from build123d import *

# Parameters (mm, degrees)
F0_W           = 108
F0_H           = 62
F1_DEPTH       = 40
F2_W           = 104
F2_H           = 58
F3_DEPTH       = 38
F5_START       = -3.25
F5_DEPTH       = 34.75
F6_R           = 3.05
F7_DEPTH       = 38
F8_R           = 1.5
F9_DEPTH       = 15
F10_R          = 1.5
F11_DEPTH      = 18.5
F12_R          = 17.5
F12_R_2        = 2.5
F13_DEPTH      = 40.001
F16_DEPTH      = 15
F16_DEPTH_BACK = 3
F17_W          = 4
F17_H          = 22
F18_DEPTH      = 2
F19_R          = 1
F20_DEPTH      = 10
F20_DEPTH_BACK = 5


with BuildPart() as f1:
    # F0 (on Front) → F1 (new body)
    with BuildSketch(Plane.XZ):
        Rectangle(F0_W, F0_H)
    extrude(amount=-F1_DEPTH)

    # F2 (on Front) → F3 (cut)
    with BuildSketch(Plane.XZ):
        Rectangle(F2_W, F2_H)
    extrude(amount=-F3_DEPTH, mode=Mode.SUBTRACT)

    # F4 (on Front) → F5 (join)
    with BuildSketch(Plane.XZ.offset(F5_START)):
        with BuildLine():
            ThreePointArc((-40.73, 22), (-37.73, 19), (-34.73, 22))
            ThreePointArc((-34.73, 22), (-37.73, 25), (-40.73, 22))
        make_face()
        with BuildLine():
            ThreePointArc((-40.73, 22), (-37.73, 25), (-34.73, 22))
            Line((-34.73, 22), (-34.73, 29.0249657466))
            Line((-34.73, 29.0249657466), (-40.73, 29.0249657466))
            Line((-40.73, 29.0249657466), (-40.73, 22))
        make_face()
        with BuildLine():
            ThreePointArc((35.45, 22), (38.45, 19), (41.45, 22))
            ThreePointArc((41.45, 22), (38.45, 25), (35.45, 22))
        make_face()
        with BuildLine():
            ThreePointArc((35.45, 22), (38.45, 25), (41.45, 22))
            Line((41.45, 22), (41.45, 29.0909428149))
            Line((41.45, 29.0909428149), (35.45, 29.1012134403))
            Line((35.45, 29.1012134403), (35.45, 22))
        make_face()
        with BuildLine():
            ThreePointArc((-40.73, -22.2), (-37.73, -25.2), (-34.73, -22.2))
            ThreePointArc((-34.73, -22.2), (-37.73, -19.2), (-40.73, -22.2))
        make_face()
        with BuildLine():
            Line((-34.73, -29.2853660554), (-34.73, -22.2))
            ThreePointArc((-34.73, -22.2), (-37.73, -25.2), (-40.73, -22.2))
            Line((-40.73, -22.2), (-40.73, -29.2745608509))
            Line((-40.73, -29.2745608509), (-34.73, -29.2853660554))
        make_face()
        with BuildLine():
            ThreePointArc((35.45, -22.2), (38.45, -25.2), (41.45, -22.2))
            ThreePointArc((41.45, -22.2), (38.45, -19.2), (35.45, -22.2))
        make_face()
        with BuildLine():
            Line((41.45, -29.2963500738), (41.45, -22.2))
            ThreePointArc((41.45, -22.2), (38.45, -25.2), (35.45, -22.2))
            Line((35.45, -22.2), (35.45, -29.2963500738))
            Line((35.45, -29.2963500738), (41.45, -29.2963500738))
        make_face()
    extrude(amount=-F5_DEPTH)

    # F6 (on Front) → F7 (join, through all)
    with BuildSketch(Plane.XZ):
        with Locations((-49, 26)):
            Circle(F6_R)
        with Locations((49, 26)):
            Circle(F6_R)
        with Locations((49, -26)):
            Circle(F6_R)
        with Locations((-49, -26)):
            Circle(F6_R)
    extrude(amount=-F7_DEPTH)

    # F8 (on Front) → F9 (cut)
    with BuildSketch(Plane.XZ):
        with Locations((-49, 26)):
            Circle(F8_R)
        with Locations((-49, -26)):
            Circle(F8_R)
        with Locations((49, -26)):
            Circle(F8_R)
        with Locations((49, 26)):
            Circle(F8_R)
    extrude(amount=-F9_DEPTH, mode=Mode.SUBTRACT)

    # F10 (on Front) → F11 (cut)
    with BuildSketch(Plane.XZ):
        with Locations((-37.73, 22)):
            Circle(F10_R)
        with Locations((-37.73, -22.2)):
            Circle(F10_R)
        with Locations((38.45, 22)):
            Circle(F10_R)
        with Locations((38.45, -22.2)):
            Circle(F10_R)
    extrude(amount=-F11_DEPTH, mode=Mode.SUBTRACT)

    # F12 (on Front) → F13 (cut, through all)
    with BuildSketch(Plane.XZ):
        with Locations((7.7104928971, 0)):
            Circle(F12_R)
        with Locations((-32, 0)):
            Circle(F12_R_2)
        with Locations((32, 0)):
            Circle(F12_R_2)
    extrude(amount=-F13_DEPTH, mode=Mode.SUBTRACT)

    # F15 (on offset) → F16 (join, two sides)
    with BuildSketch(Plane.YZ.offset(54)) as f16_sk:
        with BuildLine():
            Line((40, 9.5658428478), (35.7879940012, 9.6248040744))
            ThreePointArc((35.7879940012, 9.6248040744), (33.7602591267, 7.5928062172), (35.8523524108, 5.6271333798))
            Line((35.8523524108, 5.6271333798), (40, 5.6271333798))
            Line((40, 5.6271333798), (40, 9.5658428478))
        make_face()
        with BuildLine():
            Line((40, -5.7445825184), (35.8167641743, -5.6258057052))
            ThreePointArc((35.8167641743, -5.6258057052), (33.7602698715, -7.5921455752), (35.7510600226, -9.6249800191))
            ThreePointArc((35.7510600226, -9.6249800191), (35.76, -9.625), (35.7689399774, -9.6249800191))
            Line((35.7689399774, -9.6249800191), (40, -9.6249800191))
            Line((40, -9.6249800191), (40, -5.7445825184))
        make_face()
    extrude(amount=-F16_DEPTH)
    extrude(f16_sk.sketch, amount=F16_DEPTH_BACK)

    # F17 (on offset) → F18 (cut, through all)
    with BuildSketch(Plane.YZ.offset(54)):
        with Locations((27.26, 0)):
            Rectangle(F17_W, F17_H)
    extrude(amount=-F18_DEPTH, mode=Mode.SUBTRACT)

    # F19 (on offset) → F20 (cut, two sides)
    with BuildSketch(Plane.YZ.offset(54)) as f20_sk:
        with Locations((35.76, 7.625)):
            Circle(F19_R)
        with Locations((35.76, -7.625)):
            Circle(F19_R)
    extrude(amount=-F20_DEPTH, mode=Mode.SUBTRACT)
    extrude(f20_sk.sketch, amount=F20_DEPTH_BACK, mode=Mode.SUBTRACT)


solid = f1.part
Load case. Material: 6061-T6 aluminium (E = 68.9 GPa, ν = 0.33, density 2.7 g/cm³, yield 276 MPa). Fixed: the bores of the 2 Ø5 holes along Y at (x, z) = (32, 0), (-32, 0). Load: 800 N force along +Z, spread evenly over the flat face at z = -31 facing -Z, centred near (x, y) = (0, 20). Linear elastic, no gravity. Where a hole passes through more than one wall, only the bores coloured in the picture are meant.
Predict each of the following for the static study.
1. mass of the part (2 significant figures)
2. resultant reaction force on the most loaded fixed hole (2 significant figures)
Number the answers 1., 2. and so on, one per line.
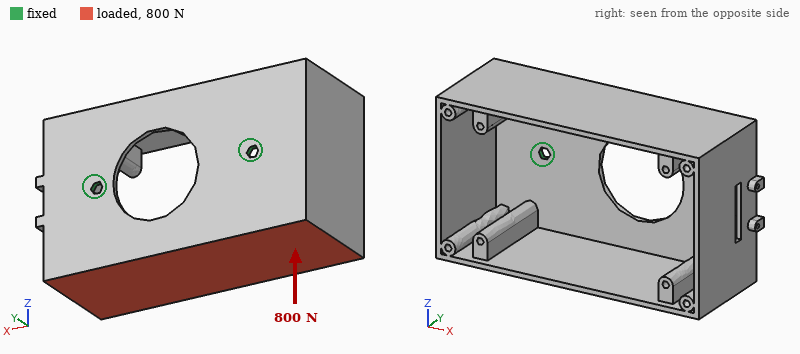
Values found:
1. 130 g
2. 440 N
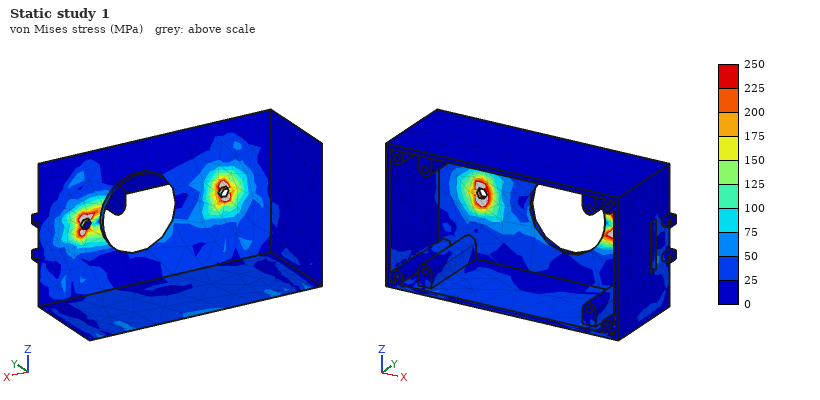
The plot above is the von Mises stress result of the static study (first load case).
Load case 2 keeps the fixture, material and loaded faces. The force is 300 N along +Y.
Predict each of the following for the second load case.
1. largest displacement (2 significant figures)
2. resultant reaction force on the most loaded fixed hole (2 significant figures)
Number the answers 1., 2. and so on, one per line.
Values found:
1. 0.62 mm
2. 160 N
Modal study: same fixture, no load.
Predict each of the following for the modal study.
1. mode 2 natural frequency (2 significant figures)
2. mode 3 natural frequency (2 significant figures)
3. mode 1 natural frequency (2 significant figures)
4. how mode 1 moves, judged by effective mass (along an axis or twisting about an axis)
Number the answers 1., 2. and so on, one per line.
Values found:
1. 630 Hz
2. 1100 Hz
3. 410 Hz
4. along Z
